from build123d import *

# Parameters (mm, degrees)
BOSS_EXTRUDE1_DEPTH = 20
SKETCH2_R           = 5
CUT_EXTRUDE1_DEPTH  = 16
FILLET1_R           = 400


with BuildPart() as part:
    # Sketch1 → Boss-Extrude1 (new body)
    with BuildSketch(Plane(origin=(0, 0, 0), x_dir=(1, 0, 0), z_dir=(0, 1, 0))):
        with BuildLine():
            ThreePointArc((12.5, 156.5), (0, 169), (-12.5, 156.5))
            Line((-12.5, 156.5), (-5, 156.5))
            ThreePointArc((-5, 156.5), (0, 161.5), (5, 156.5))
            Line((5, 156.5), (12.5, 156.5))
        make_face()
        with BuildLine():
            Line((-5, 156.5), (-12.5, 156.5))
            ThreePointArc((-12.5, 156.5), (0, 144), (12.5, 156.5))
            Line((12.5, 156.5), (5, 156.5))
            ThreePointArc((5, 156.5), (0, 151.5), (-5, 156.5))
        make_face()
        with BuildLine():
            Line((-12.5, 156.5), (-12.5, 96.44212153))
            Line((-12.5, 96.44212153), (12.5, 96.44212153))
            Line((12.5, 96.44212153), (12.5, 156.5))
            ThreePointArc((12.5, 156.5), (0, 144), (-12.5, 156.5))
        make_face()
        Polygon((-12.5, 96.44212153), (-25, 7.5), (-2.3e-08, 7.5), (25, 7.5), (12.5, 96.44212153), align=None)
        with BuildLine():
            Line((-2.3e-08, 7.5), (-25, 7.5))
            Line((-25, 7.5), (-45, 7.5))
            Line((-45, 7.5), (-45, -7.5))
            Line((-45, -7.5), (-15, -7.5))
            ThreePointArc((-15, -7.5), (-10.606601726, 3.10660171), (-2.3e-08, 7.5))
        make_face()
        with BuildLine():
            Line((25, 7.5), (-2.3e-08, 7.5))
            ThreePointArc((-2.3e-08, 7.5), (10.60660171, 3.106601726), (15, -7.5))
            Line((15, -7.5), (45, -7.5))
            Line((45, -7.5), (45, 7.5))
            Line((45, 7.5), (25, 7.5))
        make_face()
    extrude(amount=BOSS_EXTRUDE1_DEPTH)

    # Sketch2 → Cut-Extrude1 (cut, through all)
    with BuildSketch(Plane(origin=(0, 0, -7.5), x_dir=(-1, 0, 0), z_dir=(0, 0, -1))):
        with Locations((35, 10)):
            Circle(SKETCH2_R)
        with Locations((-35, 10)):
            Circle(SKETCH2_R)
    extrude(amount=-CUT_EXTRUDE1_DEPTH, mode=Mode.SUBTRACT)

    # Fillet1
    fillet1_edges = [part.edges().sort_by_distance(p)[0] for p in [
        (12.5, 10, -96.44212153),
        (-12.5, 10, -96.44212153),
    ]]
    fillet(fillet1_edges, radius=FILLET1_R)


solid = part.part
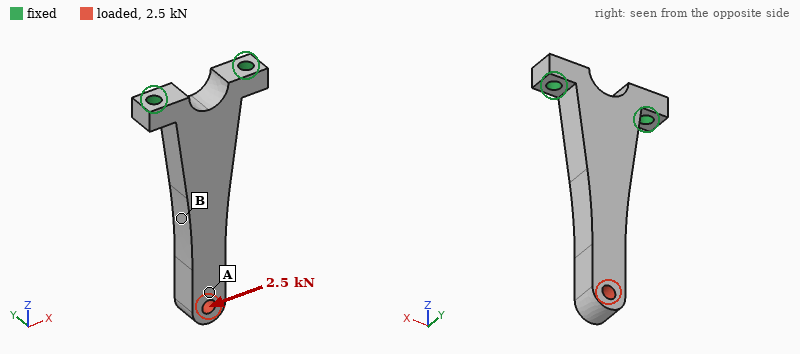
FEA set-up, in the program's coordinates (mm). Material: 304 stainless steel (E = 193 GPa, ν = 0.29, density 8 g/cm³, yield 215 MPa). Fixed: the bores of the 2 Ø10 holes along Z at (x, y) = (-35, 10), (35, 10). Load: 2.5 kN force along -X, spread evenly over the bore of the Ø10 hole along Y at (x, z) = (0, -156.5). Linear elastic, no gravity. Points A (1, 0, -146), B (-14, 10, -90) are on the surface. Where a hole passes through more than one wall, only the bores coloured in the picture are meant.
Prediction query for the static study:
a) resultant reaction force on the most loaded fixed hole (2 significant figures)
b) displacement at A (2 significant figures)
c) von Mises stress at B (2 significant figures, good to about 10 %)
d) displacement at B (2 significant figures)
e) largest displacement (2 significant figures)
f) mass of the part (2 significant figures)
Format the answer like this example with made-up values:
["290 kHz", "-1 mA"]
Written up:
["7.7 kN", "0.20 mm", "65 MPa", "0.076 mm", "0.26 mm", "950 g"]
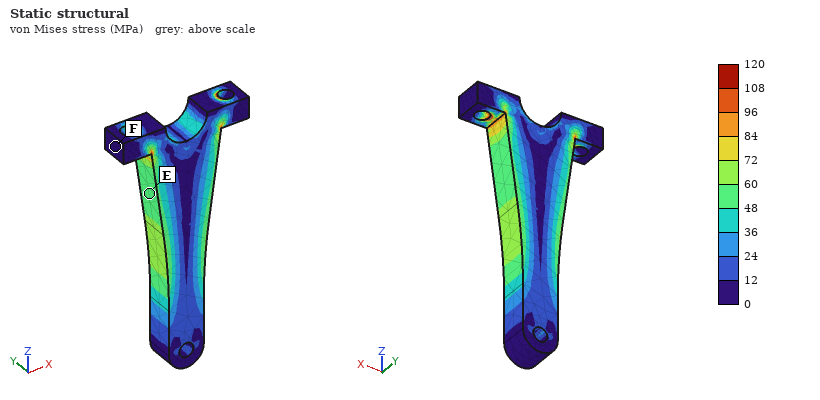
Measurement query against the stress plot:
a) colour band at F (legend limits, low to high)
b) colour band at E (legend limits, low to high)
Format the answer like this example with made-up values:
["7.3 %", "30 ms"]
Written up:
["0 to 12 MPa", "48 to 60 MPa"]
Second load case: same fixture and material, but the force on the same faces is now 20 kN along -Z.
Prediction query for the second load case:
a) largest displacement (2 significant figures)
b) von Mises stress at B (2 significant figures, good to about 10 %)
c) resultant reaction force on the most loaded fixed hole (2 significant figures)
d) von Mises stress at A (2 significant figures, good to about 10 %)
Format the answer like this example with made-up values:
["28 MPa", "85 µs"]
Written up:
["38 µm", "37 MPa", "12 kN", "38 MPa"]
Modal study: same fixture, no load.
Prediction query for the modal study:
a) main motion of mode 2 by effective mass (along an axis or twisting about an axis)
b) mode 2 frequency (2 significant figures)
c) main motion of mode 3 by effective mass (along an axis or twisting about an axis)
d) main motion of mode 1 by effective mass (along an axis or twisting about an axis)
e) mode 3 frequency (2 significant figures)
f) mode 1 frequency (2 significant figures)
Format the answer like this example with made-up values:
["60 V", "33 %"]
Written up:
["along X", "1300 Hz", "along Y", "along Y", "2900 Hz", "540 Hz"]
